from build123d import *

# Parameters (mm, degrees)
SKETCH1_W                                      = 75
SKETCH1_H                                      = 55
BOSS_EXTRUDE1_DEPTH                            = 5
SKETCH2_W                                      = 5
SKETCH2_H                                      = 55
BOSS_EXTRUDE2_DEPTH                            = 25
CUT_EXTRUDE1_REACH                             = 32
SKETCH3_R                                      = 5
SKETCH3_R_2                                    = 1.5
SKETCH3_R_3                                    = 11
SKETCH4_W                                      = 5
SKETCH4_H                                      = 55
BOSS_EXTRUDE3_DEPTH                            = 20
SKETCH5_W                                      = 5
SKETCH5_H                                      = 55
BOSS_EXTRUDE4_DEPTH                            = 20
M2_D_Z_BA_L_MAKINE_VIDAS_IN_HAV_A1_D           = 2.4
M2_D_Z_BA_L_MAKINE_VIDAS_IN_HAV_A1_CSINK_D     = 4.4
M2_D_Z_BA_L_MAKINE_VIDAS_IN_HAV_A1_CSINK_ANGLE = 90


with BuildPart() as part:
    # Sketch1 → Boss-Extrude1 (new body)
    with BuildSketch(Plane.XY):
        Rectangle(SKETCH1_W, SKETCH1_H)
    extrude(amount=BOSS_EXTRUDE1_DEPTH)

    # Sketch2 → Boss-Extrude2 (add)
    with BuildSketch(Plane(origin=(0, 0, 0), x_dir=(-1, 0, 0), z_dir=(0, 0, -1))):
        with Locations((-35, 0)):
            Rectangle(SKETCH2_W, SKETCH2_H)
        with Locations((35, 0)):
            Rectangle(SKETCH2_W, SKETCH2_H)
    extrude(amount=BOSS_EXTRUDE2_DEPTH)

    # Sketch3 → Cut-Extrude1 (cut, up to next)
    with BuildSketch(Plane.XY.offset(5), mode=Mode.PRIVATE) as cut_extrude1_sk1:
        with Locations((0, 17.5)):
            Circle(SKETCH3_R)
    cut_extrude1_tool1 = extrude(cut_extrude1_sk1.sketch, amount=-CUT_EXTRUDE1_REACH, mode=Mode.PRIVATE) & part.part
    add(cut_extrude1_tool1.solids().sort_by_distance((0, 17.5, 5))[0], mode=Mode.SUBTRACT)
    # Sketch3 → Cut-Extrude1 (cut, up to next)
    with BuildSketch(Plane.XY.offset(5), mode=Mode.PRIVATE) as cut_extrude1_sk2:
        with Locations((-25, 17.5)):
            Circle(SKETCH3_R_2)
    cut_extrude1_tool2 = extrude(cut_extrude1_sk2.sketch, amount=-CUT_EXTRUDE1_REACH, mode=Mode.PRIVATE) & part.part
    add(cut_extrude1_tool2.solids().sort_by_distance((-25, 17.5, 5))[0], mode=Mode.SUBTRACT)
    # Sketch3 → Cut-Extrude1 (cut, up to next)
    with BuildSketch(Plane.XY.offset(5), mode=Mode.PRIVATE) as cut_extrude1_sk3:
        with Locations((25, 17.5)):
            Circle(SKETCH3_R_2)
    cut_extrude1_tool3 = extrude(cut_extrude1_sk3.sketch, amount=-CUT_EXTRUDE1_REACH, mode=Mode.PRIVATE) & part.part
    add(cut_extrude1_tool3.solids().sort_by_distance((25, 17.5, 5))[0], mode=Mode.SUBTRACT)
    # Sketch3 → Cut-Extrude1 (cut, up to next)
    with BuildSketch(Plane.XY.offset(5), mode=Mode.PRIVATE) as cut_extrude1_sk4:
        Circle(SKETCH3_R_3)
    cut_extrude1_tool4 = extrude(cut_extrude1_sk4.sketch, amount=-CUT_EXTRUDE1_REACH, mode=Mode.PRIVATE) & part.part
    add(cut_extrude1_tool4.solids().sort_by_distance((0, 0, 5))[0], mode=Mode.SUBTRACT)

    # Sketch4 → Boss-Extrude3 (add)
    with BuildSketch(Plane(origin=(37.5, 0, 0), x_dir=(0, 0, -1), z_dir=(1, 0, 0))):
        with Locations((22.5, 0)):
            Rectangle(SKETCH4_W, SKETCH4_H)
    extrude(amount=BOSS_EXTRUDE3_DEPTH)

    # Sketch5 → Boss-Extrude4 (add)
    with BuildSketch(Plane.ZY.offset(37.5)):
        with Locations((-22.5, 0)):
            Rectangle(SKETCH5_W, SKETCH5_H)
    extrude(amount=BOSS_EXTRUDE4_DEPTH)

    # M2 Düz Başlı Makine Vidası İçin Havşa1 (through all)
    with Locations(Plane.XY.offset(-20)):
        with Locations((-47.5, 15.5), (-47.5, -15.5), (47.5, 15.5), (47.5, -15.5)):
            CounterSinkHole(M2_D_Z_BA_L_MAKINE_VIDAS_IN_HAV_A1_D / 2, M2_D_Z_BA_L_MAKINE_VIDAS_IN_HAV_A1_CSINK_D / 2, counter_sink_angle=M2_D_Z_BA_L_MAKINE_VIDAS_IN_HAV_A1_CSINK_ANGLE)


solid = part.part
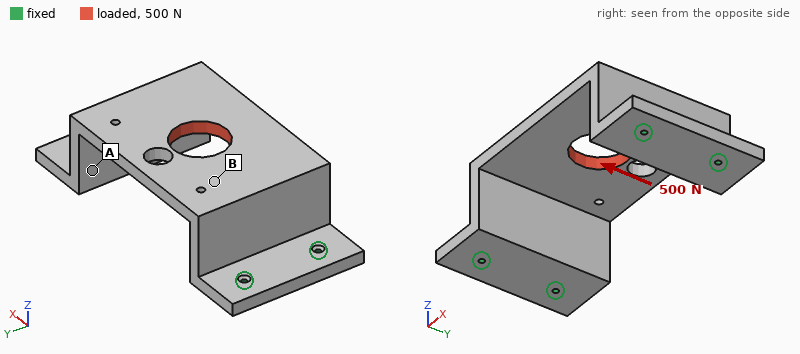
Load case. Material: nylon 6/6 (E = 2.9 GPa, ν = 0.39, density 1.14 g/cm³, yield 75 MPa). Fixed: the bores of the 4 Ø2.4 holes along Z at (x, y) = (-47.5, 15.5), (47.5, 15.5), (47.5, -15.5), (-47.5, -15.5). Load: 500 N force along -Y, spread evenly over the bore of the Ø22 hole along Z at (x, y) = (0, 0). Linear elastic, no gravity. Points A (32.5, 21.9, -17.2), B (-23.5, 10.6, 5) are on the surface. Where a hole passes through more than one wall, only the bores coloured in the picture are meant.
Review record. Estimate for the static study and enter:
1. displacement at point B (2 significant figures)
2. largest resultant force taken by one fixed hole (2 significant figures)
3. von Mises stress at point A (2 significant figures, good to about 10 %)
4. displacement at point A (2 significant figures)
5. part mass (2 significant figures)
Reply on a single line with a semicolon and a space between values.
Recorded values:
0.29 mm; 270 N; 5.3 MPa; 0.20 mm; 49 g
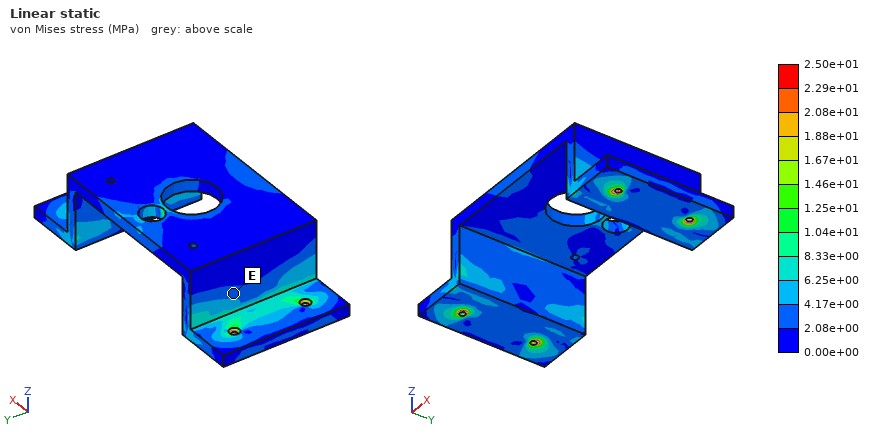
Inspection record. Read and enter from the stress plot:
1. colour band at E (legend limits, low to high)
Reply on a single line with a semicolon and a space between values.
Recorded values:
2.08e+00 to 4.17e+00 MPa
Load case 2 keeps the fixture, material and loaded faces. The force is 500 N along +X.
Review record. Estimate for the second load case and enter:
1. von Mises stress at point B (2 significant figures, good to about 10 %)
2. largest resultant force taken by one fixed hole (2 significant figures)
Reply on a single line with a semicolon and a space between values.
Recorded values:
8.1 MPa; 140 N
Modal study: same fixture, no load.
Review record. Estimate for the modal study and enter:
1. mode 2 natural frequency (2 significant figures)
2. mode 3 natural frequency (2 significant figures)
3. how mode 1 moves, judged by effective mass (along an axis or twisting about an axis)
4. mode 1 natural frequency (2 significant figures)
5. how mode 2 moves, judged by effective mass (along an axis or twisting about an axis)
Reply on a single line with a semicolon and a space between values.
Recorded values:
1200 Hz; 1300 Hz; along X; 830 Hz; along Y
